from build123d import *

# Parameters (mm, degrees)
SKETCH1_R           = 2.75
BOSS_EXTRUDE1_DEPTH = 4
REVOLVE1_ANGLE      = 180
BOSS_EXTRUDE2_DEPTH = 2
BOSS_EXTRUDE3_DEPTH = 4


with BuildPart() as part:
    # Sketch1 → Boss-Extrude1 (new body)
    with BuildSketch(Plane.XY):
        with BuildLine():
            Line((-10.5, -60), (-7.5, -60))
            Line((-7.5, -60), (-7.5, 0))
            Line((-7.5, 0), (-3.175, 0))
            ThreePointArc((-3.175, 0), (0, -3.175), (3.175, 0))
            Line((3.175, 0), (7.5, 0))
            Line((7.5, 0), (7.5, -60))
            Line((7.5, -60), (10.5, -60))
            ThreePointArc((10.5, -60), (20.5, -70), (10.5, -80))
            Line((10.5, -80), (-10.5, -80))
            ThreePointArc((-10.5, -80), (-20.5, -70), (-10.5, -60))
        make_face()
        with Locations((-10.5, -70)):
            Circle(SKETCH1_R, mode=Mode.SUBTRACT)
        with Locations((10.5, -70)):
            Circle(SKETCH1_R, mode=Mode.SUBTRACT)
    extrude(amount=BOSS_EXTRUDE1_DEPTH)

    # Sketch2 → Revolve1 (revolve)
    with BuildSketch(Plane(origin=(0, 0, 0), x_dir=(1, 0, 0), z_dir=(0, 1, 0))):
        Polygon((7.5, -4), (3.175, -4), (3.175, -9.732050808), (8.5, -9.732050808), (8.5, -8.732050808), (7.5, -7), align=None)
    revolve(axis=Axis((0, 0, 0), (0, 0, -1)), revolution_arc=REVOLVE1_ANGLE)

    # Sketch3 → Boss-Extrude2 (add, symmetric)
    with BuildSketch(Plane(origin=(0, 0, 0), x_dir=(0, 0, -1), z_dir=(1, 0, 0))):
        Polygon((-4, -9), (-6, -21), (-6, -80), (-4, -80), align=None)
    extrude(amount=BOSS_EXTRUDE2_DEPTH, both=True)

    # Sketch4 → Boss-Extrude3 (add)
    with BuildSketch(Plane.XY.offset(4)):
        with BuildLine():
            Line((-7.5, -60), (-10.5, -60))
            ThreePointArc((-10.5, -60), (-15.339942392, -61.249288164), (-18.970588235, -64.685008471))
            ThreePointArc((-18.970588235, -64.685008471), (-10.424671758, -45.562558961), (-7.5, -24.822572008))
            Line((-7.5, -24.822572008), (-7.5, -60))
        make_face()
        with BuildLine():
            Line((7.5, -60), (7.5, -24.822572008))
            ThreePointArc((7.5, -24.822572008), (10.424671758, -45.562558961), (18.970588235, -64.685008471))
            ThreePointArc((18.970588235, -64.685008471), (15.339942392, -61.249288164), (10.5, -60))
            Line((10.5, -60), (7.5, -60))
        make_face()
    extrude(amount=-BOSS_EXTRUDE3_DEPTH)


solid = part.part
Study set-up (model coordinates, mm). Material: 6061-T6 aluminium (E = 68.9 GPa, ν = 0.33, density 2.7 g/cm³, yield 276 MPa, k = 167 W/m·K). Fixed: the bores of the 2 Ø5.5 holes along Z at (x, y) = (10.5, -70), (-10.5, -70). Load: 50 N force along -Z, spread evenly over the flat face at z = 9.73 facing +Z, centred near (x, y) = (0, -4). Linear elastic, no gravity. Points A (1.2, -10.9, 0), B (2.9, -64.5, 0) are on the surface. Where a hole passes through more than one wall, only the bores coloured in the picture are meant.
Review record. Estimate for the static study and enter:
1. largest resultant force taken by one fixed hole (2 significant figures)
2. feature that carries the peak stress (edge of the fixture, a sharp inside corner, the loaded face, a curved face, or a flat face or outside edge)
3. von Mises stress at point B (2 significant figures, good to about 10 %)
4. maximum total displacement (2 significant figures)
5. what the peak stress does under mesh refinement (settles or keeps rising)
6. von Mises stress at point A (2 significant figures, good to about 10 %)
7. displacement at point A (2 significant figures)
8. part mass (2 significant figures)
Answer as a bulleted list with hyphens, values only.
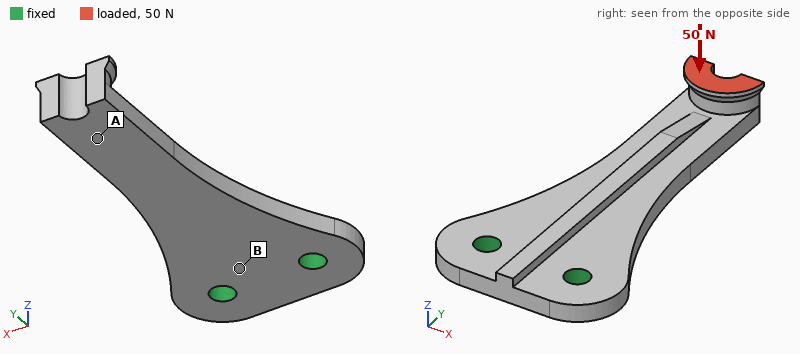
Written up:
- 35 N
- edge of the fixture
- 23 MPa
- 0.38 mm
- keeps rising
- 7.6 MPa
- 0.29 mm
- 22 g
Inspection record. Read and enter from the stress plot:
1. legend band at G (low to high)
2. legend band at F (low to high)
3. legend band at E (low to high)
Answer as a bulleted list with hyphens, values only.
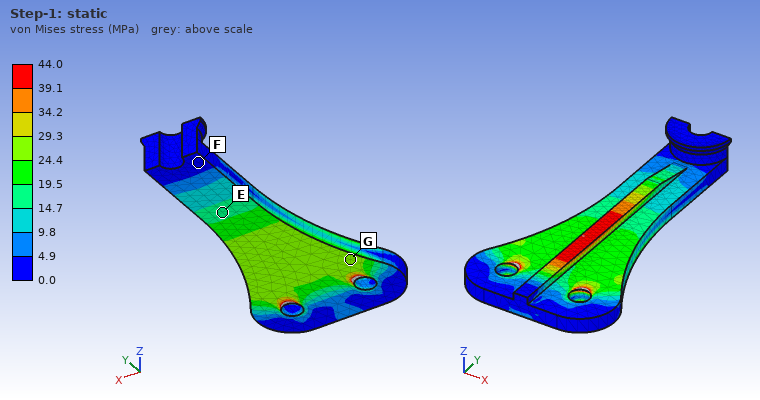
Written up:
- 24.4 to 29.3 MPa
- 0.0 to 4.9 MPa
- 14.7 to 19.5 MPa
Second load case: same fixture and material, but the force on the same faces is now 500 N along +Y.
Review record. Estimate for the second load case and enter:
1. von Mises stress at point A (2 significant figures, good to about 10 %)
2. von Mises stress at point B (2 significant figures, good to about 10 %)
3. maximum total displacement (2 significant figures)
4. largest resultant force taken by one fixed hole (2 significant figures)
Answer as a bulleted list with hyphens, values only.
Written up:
- 76 MPa
- 26 MPa
- 0.77 mm
- 250 N
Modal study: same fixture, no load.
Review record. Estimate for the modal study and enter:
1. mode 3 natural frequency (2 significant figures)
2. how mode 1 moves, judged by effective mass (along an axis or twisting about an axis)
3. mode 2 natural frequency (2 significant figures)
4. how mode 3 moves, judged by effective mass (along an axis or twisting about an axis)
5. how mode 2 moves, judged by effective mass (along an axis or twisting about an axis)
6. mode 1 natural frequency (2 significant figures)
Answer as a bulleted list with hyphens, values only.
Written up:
- 4900 Hz
- along Z
- 4000 Hz
- along Z
- along X
- 920 Hz
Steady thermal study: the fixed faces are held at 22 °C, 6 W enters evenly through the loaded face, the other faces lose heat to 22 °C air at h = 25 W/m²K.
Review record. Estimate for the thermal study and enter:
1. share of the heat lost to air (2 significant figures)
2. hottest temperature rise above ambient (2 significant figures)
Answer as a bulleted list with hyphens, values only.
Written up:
- 17 %
- 28 K
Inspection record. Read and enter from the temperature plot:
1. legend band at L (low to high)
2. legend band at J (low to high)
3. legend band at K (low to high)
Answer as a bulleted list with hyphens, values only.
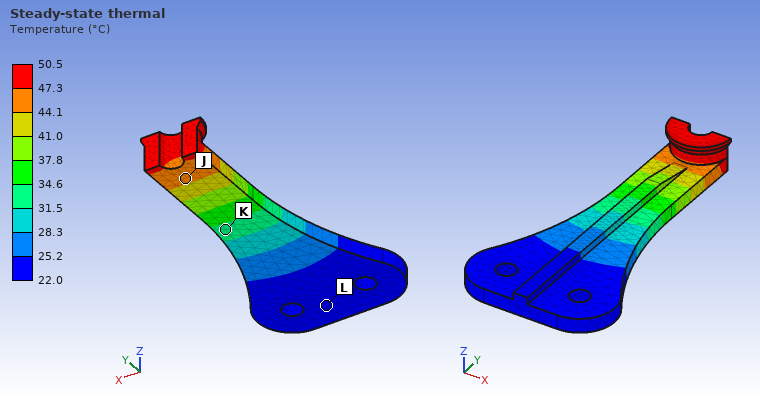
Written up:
- 22.0 to 25.2 °C
- 44.1 to 47.3 °C
- 31.5 to 34.6 °C
